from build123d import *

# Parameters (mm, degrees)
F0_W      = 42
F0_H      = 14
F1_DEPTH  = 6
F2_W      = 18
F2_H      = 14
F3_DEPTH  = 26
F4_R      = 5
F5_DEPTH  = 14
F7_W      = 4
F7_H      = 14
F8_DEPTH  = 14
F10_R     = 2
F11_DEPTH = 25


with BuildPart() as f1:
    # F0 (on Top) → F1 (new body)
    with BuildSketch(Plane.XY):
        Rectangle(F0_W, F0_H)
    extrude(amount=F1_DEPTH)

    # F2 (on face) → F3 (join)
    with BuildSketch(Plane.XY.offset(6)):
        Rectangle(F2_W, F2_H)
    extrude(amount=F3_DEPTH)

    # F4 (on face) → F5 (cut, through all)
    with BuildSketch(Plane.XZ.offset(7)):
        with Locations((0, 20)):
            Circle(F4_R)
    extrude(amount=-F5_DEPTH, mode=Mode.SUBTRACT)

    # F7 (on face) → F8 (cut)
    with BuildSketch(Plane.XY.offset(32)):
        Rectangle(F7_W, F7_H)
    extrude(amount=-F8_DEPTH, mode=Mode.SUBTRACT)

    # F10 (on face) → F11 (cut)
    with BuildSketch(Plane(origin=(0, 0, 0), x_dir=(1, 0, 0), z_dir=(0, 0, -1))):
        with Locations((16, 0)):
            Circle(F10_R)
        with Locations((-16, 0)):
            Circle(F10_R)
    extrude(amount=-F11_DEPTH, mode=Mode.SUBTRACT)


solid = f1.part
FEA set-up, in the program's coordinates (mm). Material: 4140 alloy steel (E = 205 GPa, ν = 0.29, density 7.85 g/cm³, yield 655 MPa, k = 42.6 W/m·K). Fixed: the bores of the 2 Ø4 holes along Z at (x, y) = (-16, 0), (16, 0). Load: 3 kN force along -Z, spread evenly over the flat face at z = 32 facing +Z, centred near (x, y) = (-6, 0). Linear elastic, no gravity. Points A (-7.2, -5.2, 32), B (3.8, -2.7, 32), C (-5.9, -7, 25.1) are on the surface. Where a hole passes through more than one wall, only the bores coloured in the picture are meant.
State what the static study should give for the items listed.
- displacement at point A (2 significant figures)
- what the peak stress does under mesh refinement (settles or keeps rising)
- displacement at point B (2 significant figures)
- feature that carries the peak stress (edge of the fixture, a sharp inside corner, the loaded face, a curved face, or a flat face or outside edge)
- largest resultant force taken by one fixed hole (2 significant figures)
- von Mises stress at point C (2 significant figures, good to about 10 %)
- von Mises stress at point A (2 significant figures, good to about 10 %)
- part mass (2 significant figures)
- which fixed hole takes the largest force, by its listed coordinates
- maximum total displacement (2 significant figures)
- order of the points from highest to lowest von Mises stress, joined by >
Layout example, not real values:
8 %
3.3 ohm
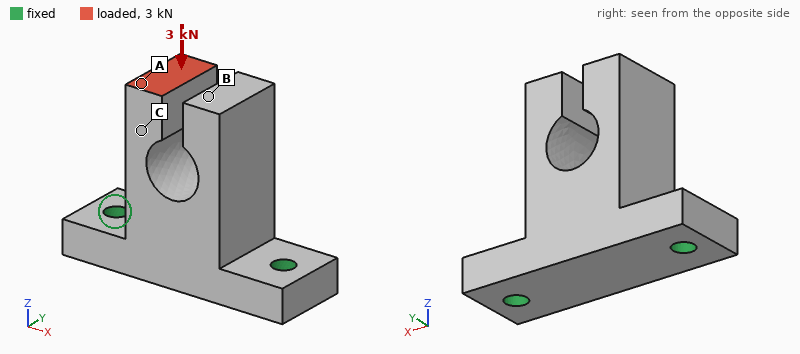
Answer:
17 µm
keeps rising
7.1 µm
edge of the fixture
2.2 kN
55 MPa
30 MPa
66 g
(-16, 0)
23 µm
C > A > B
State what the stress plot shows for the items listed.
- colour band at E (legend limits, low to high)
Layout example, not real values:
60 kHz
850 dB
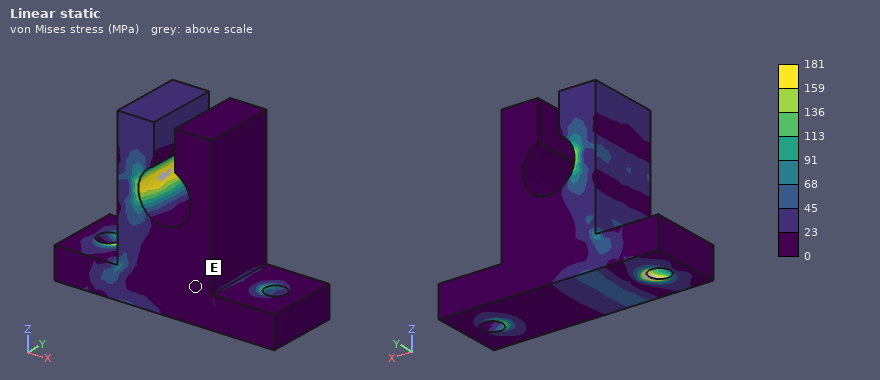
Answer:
0 to 23 MPa
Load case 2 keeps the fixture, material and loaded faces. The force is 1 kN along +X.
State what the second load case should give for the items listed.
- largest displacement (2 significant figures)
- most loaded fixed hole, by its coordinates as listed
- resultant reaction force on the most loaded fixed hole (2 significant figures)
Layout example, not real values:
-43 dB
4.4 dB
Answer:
0.10 mm
(16, 0)
1.4 kN
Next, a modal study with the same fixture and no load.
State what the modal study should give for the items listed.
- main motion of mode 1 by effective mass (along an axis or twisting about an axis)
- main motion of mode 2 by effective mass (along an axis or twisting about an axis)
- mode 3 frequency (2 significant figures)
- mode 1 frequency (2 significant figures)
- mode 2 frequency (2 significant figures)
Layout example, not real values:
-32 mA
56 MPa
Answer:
along Y
along X
8800 Hz
5200 Hz
7600 Hz
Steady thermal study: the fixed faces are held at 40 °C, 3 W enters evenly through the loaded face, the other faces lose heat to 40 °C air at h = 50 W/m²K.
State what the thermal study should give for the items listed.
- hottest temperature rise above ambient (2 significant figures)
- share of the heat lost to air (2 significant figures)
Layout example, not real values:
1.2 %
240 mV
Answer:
21 K
29 %
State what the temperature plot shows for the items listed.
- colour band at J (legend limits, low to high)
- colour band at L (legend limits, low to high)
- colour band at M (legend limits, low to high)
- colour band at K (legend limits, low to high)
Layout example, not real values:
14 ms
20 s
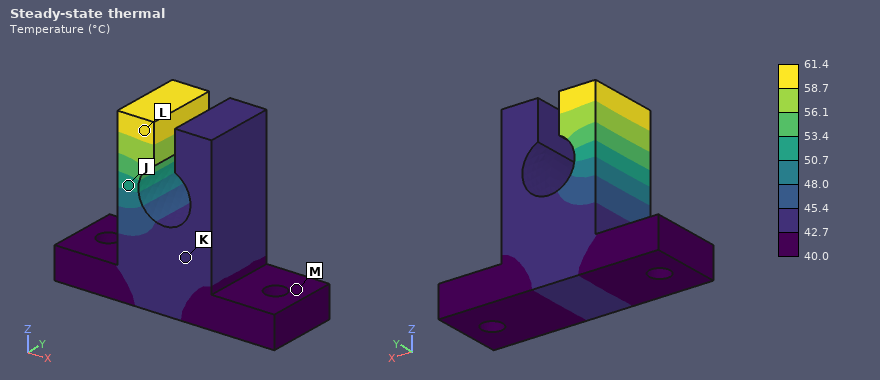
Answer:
50.7 to 53.4 °C
58.7 to 61.4 °C
40.0 to 42.7 °C
42.7 to 45.4 °C
